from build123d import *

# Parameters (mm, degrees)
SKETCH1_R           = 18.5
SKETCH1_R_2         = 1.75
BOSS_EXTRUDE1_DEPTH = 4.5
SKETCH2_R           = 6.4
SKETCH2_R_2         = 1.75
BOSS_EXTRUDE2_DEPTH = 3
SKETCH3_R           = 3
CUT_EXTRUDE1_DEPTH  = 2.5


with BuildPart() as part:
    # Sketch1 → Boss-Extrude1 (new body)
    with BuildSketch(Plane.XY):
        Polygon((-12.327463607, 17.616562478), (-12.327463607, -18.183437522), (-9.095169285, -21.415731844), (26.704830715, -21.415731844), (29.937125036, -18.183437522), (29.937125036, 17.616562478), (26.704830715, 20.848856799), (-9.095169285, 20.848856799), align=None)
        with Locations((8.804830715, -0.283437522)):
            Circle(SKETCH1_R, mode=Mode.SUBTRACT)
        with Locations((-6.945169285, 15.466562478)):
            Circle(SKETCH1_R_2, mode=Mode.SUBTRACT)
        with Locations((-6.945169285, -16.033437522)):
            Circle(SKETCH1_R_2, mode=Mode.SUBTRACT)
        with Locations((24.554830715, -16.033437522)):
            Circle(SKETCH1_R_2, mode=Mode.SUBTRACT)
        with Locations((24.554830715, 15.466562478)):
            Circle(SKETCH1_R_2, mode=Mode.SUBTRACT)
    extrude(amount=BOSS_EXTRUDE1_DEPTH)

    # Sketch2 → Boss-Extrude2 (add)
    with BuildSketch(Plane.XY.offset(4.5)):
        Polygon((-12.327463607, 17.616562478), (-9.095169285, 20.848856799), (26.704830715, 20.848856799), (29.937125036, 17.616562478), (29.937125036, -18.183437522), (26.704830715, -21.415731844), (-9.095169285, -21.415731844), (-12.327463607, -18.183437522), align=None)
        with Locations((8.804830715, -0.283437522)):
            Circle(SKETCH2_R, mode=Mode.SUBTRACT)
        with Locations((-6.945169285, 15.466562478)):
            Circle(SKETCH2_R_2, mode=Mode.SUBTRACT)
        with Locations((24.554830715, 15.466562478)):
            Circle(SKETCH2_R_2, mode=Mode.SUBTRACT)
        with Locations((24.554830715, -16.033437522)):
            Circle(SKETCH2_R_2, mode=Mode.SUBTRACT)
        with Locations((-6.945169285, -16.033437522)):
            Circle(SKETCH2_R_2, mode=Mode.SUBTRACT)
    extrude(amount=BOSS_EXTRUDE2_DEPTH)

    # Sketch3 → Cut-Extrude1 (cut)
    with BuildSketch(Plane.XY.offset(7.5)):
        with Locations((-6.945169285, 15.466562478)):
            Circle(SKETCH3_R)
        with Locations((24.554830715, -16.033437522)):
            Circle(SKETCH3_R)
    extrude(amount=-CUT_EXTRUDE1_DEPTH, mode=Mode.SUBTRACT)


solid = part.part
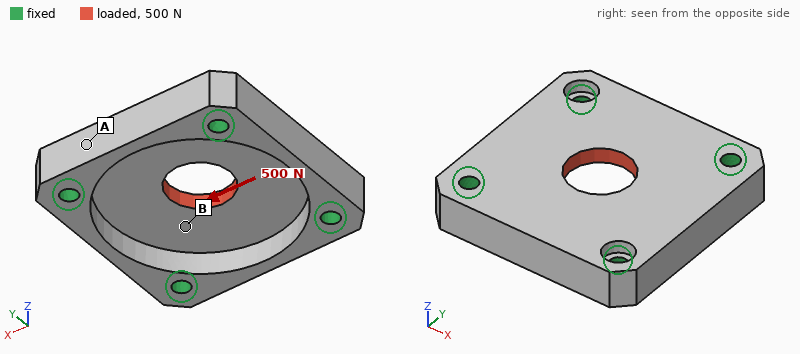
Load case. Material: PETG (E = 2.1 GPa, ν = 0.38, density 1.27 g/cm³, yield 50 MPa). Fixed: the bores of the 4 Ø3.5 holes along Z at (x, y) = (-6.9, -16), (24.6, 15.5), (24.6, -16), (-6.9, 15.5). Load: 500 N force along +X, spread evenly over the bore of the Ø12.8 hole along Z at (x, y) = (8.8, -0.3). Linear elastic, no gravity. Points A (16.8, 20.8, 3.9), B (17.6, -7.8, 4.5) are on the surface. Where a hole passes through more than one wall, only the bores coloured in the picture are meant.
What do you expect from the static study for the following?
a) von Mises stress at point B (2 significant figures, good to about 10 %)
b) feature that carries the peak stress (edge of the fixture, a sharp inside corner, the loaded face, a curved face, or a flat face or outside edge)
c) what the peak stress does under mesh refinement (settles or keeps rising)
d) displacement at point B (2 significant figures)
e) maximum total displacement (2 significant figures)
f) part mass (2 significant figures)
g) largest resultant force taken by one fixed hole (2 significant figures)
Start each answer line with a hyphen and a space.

- 4.0 MPa
- edge of the fixture
- keeps rising
- 34 µm
- 50 µm
- 9.7 g
- 150 N
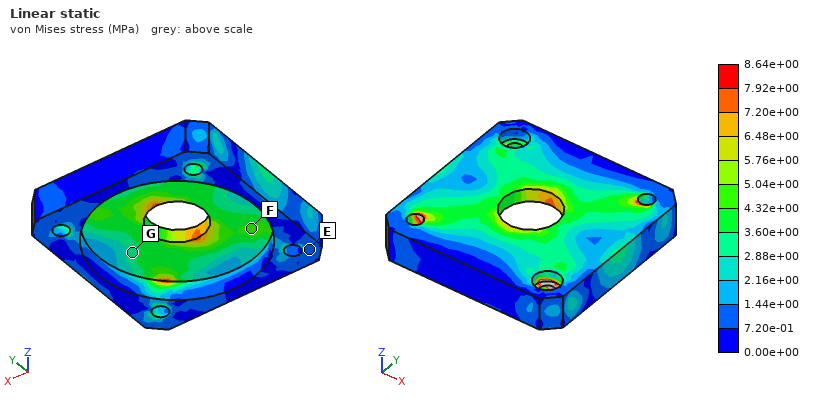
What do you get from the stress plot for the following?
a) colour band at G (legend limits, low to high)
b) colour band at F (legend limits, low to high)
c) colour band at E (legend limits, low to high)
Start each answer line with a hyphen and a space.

- 2.88e+00 to 3.60e+00 MPa
- 4.32e+00 to 5.04e+00 MPa
- 7.20e-01 to 1.44e+00 MPa
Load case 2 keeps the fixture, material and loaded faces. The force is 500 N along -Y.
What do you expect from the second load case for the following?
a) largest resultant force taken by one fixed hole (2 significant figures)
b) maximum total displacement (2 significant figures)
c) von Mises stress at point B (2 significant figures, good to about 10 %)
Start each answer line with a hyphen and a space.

- 150 N
- 50 µm
- 3.9 MPa
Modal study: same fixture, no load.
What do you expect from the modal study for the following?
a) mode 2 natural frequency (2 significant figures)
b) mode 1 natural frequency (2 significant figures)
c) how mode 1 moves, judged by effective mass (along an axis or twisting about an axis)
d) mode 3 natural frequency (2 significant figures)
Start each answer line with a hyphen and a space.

- 6200 Hz
- 4300 Hz
- along Z
- 6600 Hz
